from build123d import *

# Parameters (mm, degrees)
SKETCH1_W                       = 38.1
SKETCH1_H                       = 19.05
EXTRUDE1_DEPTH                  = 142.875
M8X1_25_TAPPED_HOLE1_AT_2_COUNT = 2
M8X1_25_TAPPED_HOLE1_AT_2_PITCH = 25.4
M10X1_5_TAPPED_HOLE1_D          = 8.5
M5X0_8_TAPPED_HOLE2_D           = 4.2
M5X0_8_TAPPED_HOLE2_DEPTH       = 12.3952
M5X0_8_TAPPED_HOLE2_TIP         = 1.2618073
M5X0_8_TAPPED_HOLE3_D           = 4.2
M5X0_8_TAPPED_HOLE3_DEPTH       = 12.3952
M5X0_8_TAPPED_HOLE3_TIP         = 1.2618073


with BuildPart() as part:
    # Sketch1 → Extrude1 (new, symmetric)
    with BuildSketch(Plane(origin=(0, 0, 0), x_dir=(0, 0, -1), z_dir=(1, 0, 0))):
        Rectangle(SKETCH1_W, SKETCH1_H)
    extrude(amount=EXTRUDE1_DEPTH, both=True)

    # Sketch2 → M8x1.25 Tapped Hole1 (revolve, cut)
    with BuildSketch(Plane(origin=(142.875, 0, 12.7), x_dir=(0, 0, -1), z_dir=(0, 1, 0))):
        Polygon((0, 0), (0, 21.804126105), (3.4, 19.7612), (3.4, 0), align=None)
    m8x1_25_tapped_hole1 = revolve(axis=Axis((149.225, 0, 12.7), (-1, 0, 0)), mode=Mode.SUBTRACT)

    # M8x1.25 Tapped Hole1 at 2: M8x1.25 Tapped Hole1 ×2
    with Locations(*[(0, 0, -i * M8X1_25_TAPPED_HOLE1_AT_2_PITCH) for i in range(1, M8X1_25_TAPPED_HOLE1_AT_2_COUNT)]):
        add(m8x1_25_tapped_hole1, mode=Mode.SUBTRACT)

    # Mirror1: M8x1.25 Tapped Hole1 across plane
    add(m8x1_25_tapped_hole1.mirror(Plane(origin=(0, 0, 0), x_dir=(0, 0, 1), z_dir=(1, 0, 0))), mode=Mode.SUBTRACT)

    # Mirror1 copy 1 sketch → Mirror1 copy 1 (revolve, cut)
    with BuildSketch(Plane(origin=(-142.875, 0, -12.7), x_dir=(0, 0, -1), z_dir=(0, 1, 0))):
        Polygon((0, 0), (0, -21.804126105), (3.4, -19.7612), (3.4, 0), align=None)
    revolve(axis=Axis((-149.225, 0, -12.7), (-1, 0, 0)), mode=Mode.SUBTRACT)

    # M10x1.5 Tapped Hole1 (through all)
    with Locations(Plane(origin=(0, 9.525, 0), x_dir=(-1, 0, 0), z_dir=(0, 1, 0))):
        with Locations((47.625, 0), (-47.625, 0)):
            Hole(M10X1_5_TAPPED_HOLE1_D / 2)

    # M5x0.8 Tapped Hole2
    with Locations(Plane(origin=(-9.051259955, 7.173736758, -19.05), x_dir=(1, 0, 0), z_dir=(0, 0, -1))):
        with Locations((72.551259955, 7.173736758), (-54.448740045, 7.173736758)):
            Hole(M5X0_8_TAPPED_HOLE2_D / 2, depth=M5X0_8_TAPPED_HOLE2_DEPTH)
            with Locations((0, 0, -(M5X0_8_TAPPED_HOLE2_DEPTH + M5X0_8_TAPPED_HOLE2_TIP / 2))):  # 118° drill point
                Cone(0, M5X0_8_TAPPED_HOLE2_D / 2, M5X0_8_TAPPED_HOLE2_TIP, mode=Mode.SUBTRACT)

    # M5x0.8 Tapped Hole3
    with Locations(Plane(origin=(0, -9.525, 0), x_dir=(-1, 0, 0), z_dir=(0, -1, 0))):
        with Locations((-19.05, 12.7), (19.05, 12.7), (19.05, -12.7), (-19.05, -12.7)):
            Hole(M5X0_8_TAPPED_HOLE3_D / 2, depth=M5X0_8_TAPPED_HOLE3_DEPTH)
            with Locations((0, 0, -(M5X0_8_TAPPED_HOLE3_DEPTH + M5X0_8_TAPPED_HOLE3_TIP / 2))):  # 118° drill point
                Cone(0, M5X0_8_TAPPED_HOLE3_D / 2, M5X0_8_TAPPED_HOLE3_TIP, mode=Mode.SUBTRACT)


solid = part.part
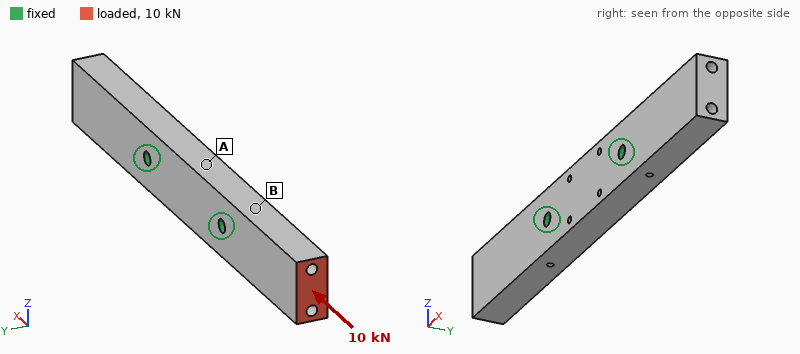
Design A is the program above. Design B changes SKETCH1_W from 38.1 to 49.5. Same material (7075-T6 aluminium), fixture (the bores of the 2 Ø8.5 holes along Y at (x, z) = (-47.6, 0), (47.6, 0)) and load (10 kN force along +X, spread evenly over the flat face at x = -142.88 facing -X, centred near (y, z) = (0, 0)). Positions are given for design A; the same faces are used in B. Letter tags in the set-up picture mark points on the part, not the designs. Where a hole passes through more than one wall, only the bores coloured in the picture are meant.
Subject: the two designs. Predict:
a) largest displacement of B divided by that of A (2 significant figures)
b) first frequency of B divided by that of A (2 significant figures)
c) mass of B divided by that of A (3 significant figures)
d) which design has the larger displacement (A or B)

0.80
0.96
1.31
A
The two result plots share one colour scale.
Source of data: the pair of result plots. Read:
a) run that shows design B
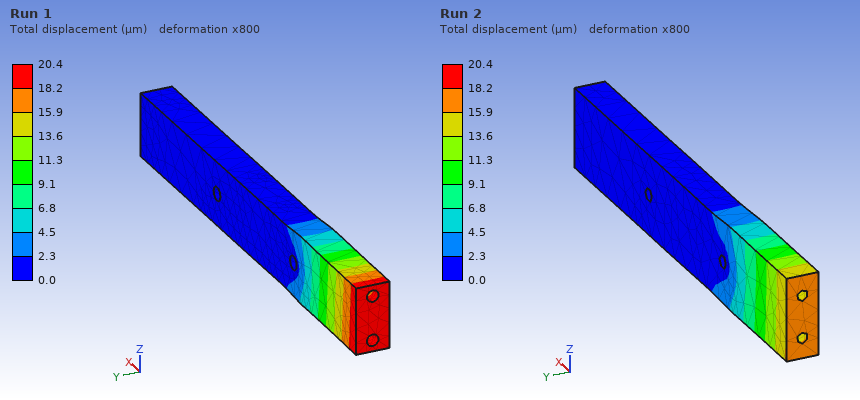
Run 2
